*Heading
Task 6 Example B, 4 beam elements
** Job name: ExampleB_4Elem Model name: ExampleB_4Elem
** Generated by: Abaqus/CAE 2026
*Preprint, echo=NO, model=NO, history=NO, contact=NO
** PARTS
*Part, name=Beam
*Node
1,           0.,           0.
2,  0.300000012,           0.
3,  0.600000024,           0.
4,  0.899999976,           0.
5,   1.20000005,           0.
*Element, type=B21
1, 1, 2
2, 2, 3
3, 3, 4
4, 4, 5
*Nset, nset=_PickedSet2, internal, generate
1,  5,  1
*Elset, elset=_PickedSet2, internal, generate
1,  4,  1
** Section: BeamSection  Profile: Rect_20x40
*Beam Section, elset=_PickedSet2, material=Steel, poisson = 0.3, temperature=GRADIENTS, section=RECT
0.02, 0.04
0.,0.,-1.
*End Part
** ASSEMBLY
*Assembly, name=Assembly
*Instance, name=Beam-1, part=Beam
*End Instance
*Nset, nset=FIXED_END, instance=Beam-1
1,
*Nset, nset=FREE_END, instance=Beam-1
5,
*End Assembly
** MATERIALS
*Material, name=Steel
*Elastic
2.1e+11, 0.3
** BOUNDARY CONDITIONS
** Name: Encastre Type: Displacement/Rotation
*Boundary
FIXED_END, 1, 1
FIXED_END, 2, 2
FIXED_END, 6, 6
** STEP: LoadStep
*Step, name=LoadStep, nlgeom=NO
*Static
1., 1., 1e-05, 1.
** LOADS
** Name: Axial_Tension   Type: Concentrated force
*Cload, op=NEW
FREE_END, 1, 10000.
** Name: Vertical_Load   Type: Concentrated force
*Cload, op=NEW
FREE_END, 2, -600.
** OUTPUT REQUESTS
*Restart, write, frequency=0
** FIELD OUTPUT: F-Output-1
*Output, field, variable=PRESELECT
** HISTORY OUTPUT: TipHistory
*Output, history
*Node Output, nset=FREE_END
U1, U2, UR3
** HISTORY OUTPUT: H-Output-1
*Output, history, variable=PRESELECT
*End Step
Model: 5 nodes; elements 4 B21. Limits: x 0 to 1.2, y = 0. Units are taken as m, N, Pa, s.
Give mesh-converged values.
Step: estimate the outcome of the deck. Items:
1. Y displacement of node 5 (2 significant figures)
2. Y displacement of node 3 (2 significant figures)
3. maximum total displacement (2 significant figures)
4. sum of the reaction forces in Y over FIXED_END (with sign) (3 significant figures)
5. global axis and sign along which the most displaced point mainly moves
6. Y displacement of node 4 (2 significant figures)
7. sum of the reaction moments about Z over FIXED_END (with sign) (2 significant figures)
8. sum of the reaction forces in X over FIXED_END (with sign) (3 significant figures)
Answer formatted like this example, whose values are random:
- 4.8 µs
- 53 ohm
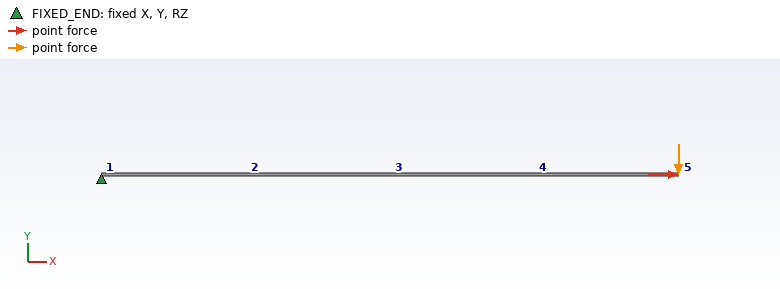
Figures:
- -0.015 m
- -0.0048 m
- 0.015 m
- 600 N
- -Y
- -0.0098 m
- 720 N·m
- -10000 N
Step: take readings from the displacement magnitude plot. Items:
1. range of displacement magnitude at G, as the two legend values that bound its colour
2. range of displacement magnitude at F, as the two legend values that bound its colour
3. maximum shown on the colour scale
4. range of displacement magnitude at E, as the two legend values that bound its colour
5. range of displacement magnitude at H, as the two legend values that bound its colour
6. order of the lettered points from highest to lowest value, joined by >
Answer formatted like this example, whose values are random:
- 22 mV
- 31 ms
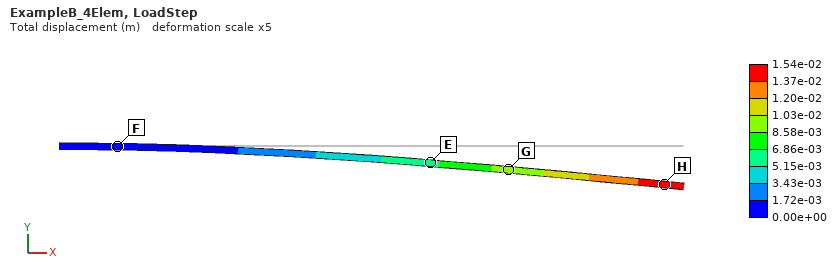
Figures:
- 8.58e-03 to 1.03e-02 m
- 0.00e+00 to 1.72e-03 m
- 1.54e-02 m
- 5.15e-03 to 6.86e-03 m
- 1.37e-02 to 1.54e-02 m
- H > G > E > F
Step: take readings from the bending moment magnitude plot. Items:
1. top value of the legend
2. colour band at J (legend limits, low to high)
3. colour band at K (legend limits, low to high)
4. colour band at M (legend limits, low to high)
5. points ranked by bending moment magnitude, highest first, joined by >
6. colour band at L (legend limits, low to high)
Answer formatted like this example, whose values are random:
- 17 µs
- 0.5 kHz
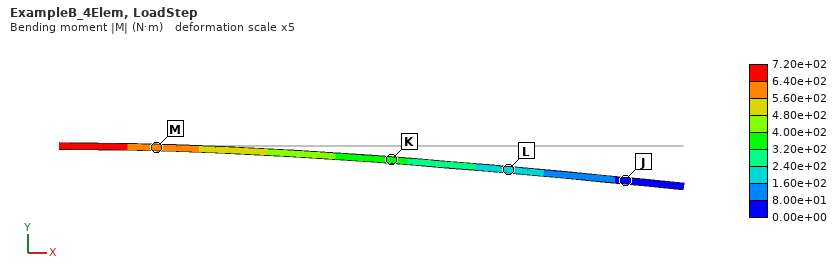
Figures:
- 7.20e+02 N·m
- 0.00e+00 to 8.00e+01 N·m
- 3.20e+02 to 4.00e+02 N·m
- 5.60e+02 to 6.40e+02 N·m
- M > K > L > J
- 1.60e+02 to 2.40e+02 N·m
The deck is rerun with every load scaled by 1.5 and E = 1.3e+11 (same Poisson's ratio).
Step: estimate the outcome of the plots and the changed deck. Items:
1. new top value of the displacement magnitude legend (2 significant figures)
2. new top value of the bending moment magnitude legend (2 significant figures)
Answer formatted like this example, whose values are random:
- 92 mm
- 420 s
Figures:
- 0.037 m
- 1100 N·m
